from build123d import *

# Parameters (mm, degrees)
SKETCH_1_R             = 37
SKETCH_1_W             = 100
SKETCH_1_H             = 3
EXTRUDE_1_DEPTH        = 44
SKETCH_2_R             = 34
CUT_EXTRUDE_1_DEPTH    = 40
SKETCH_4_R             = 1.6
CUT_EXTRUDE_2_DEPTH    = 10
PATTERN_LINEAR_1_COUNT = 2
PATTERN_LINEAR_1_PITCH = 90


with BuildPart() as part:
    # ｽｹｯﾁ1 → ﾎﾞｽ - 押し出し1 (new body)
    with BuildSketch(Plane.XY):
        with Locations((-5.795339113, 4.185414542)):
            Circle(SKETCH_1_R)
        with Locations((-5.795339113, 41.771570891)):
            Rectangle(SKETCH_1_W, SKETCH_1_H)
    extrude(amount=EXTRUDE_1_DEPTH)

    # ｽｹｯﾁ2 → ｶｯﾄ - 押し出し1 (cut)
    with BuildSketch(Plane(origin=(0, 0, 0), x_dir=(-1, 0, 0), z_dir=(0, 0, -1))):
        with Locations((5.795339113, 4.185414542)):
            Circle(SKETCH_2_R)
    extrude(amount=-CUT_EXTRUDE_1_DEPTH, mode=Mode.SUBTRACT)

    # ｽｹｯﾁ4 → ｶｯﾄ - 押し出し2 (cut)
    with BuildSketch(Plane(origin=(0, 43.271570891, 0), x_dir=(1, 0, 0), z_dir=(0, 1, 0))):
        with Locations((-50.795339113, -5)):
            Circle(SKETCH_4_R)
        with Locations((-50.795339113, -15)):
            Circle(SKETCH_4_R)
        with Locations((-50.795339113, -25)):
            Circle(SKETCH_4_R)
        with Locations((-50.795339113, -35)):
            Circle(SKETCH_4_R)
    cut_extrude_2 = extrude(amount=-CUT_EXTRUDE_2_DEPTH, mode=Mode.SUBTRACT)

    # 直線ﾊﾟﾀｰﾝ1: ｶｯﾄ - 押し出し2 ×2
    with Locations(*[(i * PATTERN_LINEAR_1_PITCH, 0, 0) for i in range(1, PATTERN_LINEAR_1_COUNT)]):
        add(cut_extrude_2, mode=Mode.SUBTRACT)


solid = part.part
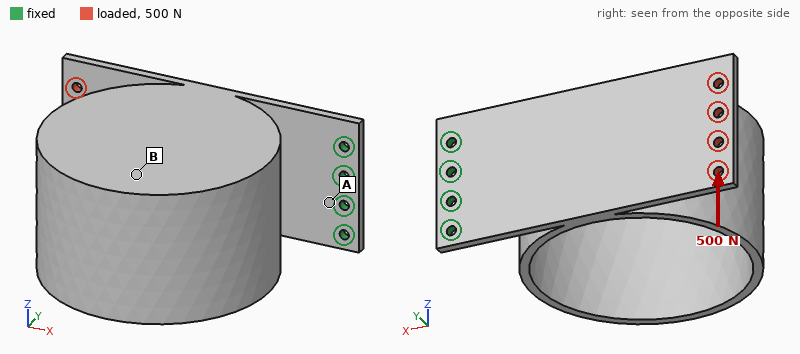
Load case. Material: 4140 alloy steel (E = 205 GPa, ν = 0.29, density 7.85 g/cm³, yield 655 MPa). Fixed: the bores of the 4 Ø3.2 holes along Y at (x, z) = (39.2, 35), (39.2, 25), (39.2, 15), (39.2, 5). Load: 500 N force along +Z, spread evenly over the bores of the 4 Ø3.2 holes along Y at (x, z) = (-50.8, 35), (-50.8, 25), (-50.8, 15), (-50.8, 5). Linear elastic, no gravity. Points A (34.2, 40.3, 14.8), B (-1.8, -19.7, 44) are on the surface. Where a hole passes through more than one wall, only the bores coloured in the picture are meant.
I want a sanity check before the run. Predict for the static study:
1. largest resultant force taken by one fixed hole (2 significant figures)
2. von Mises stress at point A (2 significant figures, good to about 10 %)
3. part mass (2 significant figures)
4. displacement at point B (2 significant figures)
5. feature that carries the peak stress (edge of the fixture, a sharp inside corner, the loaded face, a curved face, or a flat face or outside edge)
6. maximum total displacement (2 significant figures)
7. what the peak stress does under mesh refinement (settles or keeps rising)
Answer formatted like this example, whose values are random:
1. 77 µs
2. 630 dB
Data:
1. 1.4 kN
2. 18 MPa
3. 440 g
4. 13 µm
5. edge of the fixture
6. 39 µm
7. keeps rising
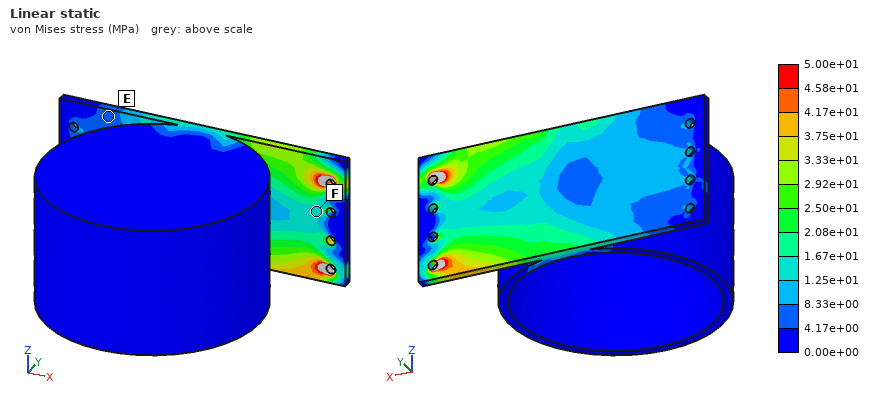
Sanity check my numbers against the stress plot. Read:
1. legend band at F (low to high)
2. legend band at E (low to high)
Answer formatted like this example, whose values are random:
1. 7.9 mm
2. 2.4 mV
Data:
1. 1.25e+01 to 1.67e+01 MPa
2. 4.17e+00 to 8.33e+00 MPa
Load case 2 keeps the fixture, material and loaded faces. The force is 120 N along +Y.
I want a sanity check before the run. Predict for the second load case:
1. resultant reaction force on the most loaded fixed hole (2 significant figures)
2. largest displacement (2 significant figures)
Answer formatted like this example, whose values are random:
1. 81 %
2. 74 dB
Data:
1. 82 N
2. 1.3 mm
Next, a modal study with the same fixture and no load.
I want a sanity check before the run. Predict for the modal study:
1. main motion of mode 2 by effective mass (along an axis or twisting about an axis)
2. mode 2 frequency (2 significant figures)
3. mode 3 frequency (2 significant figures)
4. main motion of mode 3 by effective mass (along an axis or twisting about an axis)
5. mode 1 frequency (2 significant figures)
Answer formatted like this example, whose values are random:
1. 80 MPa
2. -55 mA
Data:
1. along Z
2. 220 Hz
3. 550 Hz
4. along Y
5. 110 Hz
